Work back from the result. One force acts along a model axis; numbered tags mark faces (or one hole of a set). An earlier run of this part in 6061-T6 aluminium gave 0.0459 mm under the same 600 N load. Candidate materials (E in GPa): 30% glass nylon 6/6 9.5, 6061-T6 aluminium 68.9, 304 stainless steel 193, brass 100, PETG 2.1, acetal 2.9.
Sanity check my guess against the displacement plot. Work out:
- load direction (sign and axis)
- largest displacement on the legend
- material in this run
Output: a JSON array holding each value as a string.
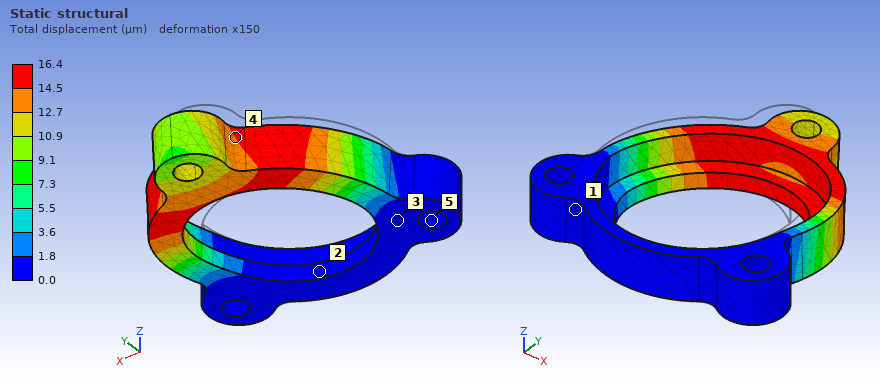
["+X", "16.4 µm", "304 stainless steel"]
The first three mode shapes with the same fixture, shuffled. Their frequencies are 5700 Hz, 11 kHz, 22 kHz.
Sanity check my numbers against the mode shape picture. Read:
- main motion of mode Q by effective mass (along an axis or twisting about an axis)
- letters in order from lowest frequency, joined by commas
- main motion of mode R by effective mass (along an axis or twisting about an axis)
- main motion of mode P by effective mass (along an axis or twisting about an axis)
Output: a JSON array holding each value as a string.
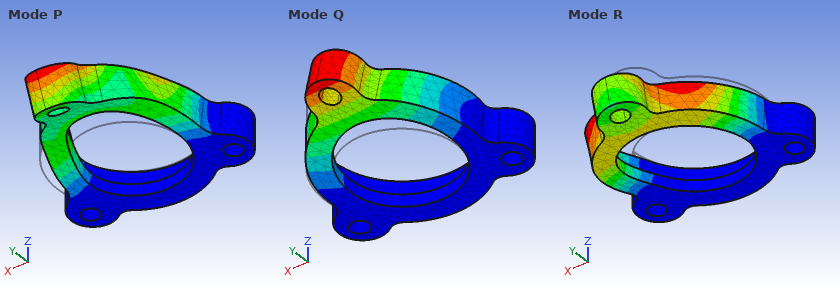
["along Z", "Q, R, P", "along X", "along Y"]
